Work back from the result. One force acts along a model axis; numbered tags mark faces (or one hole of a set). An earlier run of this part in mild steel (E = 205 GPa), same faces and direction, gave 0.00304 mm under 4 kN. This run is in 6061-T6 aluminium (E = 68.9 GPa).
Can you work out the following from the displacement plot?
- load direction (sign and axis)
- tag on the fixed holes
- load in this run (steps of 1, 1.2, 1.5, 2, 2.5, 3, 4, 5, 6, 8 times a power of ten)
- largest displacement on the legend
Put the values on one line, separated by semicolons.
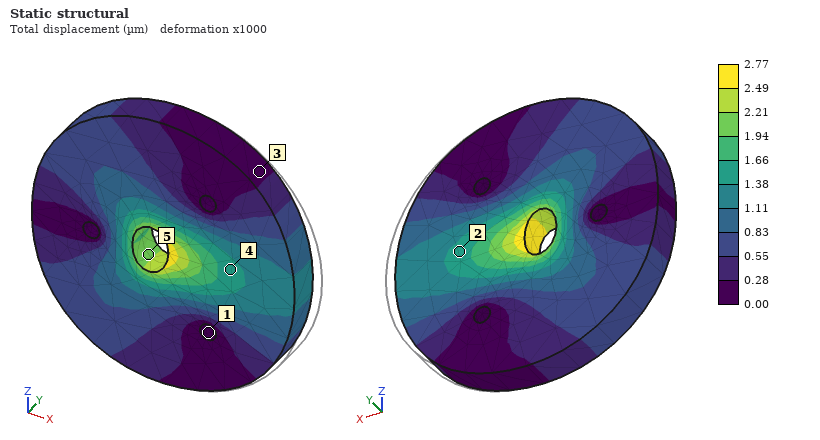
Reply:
-X; 1; 1.2 kN; 2.77 µm
